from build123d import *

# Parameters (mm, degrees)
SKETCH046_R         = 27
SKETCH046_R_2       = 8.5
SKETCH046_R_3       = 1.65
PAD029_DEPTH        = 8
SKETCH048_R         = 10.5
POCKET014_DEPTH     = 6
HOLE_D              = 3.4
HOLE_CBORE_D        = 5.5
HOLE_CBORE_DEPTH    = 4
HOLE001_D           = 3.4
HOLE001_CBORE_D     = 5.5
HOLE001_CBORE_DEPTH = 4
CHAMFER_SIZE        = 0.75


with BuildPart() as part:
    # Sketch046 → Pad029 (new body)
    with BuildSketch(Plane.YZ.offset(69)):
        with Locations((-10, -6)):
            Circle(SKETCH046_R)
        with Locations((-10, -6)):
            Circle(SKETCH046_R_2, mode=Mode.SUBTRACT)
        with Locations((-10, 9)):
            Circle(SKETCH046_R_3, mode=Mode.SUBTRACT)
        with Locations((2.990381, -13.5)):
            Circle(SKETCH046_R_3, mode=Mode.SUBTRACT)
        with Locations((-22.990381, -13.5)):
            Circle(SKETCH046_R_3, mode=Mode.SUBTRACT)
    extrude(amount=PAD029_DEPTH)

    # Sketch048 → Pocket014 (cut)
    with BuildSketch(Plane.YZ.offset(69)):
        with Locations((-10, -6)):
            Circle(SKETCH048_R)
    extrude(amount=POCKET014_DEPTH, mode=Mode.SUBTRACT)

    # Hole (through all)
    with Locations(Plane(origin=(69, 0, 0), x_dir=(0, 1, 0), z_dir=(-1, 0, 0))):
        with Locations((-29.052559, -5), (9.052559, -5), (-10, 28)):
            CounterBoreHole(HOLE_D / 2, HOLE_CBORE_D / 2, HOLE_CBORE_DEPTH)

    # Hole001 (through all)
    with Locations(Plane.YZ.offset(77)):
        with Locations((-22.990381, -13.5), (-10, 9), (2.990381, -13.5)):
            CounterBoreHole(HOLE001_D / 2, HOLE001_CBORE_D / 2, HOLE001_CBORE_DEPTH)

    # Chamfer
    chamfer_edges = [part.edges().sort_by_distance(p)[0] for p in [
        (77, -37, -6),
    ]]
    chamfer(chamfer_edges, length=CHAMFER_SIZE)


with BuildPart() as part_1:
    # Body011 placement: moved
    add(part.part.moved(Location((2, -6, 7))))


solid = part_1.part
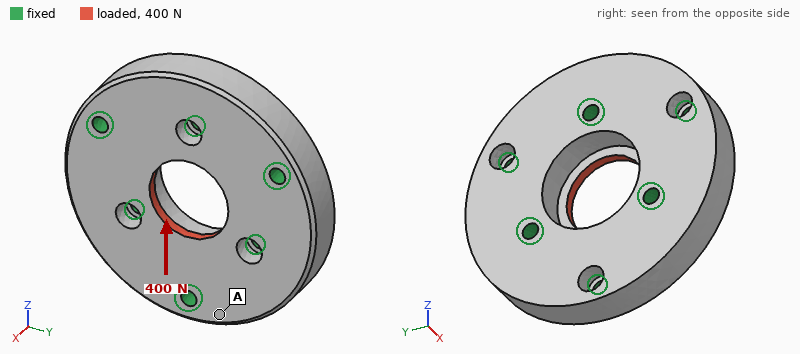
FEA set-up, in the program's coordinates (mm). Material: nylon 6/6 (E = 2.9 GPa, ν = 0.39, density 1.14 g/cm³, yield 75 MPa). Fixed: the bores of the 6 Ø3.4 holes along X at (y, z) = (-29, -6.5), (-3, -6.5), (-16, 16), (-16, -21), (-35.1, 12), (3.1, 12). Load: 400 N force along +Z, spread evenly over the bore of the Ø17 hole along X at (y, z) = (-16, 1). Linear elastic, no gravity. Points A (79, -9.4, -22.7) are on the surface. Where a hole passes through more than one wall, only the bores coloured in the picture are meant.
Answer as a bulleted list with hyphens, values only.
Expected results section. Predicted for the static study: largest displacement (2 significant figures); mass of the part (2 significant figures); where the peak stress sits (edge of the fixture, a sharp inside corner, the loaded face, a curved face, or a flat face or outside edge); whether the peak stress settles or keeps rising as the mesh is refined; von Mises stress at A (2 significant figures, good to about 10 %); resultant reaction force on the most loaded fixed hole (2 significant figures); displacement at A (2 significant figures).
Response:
- 25 µm
- 17 g
- edge of the fixture
- keeps rising
- 0.71 MPa
- 80 N
- 3.8 µm
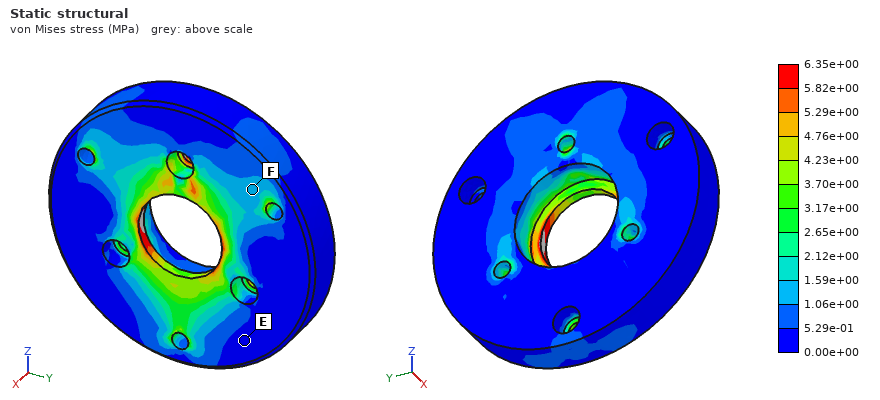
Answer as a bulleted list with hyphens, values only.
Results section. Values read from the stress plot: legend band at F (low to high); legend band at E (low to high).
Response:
- 1.06e+00 to 1.59e+00 MPa
- 0.00e+00 to 5.29e-01 MPa
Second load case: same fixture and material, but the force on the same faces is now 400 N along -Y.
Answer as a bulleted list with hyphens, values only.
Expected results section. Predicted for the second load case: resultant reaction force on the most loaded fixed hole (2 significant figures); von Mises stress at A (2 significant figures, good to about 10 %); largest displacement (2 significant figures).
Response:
- 76 N
- 0.78 MPa
- 23 µm
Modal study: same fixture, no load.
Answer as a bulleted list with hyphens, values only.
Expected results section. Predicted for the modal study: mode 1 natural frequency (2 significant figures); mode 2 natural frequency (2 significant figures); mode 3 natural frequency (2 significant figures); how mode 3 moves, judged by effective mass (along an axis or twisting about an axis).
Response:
- 7400 Hz
- 7400 Hz
- 8000 Hz
- along X
